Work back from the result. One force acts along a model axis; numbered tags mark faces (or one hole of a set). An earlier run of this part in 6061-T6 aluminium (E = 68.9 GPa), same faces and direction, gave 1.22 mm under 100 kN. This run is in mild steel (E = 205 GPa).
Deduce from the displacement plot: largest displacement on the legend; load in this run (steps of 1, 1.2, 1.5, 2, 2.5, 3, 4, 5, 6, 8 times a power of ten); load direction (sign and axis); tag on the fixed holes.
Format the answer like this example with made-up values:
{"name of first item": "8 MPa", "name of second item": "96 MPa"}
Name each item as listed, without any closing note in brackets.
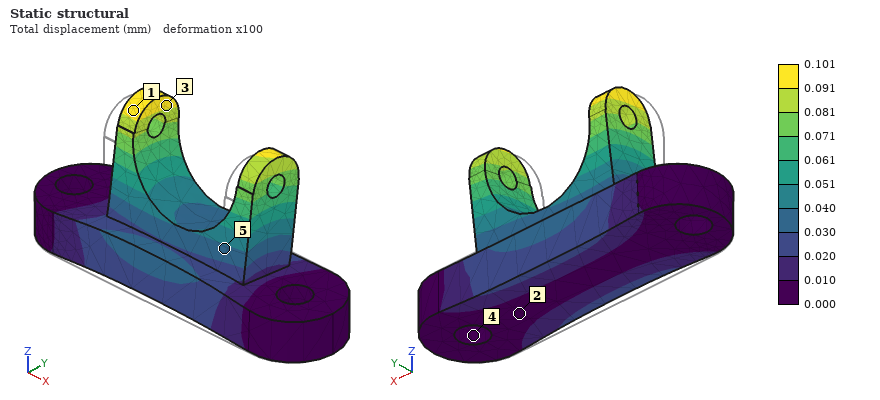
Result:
{"largest displacement on the legend": "0.101 mm", "load in this run": "25 kN", "load direction": "+Y", "tag on the fixed holes": "4"}
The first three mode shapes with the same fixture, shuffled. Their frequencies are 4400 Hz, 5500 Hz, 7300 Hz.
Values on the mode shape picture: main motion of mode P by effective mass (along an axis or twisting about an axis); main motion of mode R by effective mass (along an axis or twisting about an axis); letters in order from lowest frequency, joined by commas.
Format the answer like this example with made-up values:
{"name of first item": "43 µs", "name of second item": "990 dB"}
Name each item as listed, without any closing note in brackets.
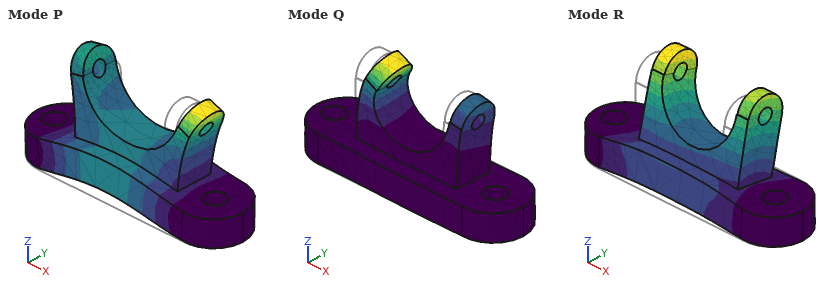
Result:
{"main motion of mode P by effective mass": "along Z", "main motion of mode R by effective mass": "along Y", "letters in order from lowest frequency, joined by commas": "R, P, Q"}
